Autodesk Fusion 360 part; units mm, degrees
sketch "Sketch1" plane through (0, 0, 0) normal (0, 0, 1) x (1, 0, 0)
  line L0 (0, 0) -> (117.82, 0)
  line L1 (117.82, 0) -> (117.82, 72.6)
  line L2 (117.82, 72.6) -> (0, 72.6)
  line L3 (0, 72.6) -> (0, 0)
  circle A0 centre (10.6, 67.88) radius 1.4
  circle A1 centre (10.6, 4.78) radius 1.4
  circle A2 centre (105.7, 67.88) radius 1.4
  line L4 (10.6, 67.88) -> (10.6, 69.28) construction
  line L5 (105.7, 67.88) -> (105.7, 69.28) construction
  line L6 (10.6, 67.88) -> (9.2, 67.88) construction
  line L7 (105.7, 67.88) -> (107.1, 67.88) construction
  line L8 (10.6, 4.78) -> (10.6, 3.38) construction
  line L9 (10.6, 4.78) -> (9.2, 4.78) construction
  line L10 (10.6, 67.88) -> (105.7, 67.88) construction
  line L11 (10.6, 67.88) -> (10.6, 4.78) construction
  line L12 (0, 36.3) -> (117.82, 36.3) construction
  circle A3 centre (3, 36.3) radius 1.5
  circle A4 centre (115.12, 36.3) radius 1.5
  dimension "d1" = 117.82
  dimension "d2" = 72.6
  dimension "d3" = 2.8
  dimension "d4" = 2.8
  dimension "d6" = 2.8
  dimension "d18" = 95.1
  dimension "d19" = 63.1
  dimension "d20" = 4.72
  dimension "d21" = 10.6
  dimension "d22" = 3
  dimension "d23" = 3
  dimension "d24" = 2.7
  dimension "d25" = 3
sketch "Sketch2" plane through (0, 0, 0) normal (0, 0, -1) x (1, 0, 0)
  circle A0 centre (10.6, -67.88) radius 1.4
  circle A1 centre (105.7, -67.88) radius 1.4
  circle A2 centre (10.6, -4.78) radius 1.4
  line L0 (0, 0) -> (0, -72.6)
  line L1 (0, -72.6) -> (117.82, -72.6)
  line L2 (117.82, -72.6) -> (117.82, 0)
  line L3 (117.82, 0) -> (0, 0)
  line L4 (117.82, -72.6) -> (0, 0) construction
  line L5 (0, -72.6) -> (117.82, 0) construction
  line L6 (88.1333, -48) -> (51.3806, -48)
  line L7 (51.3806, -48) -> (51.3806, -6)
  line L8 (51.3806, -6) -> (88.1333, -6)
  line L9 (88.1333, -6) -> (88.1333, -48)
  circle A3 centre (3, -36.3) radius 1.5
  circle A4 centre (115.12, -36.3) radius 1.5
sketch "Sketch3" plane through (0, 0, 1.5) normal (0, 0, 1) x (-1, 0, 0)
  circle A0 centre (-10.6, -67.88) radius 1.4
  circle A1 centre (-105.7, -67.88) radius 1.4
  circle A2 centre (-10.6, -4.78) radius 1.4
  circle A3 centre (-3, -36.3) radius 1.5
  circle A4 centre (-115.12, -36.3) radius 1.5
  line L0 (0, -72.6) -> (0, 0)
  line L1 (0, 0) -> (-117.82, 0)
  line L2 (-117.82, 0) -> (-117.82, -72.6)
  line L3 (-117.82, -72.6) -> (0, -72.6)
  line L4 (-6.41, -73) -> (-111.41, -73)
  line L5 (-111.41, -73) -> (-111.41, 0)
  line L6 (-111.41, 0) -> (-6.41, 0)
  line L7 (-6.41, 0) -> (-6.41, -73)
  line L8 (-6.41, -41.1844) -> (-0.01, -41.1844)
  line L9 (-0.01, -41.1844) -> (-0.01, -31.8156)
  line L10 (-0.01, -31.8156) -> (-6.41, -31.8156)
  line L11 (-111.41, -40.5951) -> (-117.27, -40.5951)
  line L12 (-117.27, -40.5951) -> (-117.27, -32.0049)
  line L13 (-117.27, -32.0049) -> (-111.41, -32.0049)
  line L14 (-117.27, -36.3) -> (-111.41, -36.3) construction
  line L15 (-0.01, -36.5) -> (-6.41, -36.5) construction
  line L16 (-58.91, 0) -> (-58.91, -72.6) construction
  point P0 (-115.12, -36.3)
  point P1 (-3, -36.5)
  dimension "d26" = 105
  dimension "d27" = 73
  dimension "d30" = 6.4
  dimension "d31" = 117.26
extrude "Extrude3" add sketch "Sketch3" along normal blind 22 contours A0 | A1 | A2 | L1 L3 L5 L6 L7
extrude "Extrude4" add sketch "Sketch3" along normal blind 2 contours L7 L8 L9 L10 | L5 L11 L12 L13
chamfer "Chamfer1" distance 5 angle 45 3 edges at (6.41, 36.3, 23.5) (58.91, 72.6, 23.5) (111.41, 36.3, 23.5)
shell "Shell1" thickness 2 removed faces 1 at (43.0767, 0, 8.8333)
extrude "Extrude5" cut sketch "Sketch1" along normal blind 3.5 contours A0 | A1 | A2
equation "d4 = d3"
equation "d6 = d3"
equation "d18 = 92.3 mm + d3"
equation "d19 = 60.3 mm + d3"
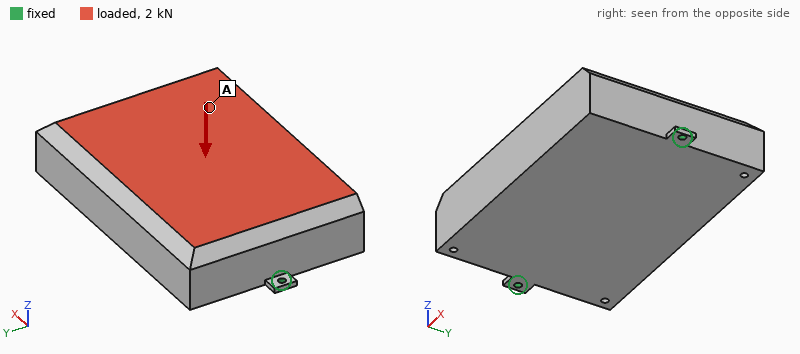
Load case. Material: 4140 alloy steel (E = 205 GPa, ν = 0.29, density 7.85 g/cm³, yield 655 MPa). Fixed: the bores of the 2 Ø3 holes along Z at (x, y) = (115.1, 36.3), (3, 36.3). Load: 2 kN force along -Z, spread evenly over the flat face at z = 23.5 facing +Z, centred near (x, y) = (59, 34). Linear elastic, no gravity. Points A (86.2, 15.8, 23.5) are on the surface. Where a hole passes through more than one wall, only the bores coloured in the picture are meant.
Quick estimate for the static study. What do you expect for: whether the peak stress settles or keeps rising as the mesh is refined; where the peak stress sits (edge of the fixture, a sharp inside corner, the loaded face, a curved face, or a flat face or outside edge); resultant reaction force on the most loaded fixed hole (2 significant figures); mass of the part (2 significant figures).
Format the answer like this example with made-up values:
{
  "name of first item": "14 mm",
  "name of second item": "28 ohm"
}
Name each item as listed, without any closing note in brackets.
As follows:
{
  "whether the peak stress settles or keeps rising as the mesh is refined": "keeps rising",
  "where the peak stress sits": "edge of the fixture",
  "resultant reaction force on the most loaded fixed hole": "1.2 kN",
  "mass of the part": "1.3 kg"
}
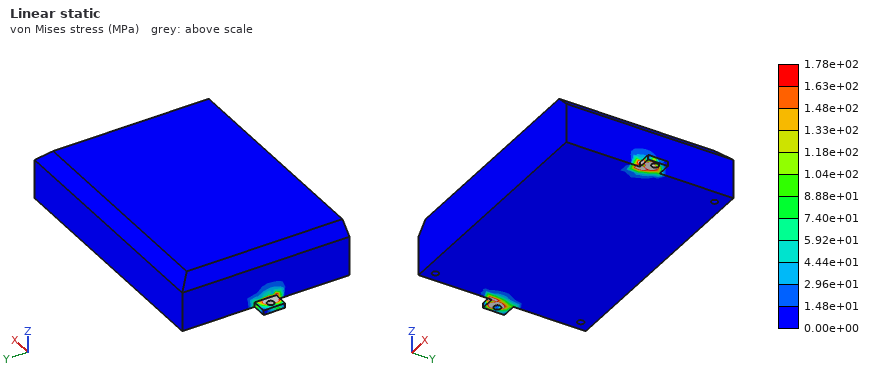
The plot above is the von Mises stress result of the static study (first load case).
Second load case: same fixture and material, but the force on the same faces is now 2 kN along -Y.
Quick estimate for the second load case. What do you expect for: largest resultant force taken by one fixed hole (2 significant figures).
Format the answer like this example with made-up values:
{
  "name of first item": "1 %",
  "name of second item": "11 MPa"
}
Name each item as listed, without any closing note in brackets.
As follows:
{
  "largest resultant force taken by one fixed hole": "1.0 kN"
}
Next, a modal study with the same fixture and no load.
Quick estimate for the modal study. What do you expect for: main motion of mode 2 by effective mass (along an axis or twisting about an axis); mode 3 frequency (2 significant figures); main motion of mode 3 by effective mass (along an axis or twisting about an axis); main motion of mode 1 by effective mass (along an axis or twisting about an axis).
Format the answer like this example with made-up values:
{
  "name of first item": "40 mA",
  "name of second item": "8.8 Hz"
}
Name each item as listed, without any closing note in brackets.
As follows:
{
  "main motion of mode 2 by effective mass": "along Z",
  "mode 3 frequency": "3200 Hz",
  "main motion of mode 3 by effective mass": "along Y",
  "main motion of mode 1 by effective mass": "along Y"
}
